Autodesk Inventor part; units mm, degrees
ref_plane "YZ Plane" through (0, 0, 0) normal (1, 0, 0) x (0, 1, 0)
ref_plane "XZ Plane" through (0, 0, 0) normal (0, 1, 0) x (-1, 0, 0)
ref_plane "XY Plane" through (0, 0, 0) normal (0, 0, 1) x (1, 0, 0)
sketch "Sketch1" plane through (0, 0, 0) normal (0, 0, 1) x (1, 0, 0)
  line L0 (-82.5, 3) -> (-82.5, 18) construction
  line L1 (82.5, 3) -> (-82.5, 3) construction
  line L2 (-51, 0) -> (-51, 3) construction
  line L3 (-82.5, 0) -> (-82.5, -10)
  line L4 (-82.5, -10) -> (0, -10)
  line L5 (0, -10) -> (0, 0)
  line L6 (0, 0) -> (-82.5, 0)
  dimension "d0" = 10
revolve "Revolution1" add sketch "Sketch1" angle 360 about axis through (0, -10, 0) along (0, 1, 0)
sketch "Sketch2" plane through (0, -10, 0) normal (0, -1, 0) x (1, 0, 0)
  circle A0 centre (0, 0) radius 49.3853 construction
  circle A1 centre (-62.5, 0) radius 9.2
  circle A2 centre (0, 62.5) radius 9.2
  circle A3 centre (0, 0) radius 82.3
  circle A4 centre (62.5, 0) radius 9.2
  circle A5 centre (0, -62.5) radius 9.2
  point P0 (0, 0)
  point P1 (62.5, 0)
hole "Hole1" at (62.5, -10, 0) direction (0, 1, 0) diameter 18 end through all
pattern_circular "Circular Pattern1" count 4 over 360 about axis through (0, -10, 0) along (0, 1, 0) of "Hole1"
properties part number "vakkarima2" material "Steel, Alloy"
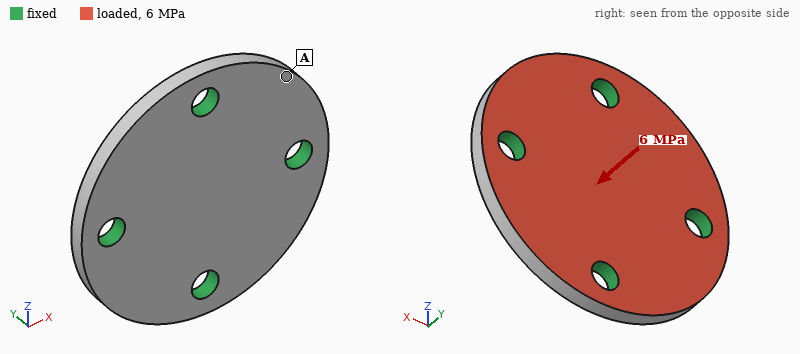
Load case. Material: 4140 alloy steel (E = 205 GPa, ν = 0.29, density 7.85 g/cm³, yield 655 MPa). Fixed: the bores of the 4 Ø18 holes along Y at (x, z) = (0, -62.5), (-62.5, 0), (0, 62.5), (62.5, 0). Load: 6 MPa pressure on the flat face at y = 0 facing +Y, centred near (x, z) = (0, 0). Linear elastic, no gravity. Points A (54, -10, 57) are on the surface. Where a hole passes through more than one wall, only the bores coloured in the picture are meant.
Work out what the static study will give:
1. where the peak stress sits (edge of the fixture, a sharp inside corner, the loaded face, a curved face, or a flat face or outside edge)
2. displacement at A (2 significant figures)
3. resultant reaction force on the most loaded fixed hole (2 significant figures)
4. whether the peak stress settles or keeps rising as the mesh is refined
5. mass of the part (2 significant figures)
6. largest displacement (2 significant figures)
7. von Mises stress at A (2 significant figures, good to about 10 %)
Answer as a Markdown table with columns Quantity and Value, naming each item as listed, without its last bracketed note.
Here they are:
| Quantity | Value |
|---|---|
| where the peak stress sits | edge of the fixture |
| displacement at A | 90 µm |
| resultant reaction force on the most loaded fixed hole | 31 kN |
| whether the peak stress settles or keeps rising as the mesh is refined | keeps rising |
| mass of the part | 1.6 kg |
| largest displacement | 97 µm |
| von Mises stress at A | 93 MPa |
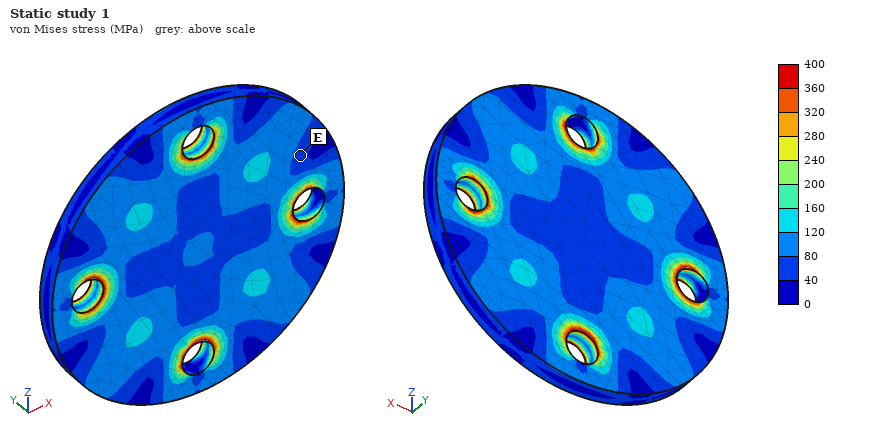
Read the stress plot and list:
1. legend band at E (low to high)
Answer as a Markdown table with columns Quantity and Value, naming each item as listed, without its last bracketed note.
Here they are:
| Quantity | Value |
|---|---|
| legend band at E | 40 to 80 MPa |
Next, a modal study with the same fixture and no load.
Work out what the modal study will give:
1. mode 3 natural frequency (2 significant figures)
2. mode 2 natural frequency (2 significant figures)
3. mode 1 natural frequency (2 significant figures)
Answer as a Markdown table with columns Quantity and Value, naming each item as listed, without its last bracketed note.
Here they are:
| Quantity | Value |
|---|---|
| mode 3 natural frequency | 5600 Hz |
| mode 2 natural frequency | 5600 Hz |
| mode 1 natural frequency | 5500 Hz |
